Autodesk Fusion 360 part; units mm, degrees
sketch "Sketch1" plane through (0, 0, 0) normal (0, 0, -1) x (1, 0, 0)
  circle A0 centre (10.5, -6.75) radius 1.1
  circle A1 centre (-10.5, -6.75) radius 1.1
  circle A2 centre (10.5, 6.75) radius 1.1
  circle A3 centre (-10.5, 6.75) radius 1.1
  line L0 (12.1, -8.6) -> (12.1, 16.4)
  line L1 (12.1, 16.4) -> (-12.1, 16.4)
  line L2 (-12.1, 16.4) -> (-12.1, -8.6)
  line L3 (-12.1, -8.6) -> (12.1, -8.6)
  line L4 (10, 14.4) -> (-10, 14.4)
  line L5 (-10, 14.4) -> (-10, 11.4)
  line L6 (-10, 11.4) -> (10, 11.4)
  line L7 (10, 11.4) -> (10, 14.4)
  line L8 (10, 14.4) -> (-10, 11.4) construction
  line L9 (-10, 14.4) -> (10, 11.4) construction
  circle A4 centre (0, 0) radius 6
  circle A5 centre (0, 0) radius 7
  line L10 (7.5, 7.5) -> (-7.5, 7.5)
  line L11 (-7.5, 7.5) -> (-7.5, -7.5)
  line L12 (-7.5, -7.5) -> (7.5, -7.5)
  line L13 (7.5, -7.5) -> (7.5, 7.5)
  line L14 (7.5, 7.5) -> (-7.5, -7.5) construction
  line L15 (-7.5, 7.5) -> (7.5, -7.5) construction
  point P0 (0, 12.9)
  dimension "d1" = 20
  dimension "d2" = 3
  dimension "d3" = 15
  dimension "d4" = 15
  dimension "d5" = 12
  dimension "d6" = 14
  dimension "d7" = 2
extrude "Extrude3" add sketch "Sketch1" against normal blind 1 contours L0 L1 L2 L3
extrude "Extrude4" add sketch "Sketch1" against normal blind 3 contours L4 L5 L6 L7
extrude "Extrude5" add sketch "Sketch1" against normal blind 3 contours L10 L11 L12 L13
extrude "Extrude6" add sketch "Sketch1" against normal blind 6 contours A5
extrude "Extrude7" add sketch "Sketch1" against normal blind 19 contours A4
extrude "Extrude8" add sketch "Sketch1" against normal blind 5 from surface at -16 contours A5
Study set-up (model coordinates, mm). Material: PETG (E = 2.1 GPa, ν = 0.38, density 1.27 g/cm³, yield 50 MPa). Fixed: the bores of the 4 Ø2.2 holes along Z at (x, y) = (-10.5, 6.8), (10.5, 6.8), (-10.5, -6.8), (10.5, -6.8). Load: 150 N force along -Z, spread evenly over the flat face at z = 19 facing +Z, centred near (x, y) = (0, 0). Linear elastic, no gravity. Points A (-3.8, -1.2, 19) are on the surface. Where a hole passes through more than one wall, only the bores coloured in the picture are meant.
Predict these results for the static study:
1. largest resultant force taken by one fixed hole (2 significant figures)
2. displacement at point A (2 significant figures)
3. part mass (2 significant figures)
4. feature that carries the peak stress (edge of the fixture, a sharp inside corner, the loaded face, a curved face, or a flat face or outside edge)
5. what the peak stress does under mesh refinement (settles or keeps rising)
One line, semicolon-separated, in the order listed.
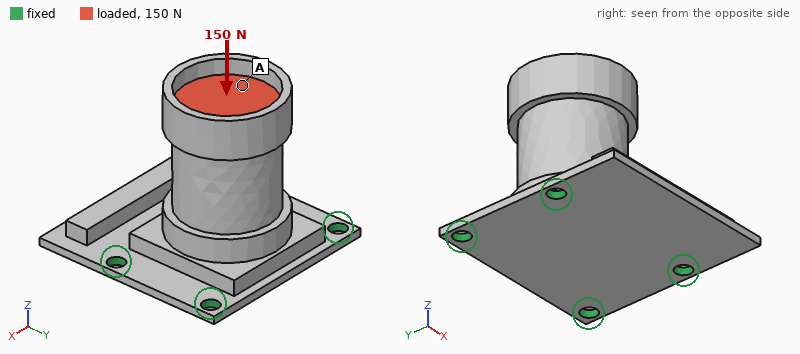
49 N; 0.15 mm; 4.2 g; edge of the fixture; keeps rising
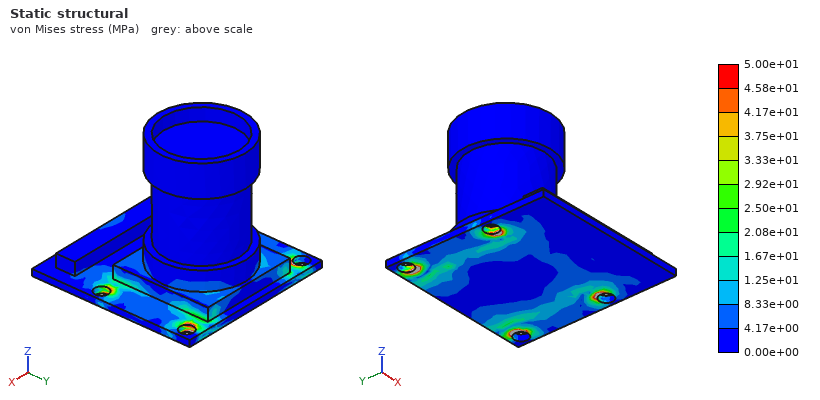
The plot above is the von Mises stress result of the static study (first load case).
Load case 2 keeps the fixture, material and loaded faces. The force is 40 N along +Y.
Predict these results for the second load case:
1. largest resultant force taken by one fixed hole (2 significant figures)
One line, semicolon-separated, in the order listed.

37 N
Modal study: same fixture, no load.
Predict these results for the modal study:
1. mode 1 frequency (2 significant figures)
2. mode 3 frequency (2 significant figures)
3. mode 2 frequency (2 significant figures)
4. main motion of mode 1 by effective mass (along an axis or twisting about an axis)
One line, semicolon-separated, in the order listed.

1500 Hz; 2100 Hz; 2100 Hz; along Y
